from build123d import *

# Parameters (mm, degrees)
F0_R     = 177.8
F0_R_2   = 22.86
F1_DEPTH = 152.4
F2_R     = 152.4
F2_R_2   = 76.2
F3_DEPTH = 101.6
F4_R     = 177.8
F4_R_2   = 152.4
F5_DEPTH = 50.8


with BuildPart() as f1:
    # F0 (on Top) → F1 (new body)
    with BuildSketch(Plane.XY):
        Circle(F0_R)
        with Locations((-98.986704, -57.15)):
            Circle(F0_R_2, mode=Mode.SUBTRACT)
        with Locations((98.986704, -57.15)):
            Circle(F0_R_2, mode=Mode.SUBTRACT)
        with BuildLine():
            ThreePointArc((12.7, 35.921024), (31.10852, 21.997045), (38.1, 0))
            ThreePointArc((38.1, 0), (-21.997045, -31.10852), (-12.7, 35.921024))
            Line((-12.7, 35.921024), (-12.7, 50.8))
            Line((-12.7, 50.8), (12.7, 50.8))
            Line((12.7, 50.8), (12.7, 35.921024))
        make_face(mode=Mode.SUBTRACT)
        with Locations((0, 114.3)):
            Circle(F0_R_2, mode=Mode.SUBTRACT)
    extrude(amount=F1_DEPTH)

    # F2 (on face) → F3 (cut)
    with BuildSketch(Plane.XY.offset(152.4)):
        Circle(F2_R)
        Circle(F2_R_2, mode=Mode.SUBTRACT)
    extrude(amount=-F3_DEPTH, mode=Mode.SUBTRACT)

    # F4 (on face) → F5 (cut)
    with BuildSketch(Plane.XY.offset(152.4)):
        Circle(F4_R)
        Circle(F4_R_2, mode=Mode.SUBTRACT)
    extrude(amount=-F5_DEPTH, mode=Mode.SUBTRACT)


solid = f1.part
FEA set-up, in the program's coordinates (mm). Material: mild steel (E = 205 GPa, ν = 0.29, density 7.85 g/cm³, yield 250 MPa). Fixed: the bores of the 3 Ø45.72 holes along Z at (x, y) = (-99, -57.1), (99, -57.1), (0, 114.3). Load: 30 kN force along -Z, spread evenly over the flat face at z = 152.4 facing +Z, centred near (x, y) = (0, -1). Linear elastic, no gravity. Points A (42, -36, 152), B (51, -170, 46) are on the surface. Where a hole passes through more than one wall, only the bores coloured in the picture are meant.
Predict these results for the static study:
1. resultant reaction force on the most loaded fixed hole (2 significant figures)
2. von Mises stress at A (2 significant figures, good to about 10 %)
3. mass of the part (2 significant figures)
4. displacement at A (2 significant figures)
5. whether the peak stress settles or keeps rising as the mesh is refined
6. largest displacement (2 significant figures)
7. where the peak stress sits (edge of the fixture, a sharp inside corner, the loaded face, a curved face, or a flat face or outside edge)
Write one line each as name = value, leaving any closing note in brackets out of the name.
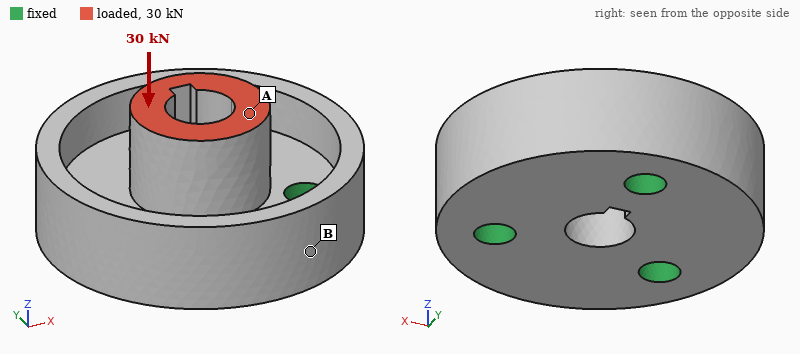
resultant reaction force on the most loaded fixed hole = 10 kN
von Mises stress at A = 2.4 MPa
mass of the part = 57 kg
displacement at A = 2.5 µm
whether the peak stress settles or keeps rising as the mesh is refined = keeps rising
largest displacement = 2.6 µm
where the peak stress sits = edge of the fixture
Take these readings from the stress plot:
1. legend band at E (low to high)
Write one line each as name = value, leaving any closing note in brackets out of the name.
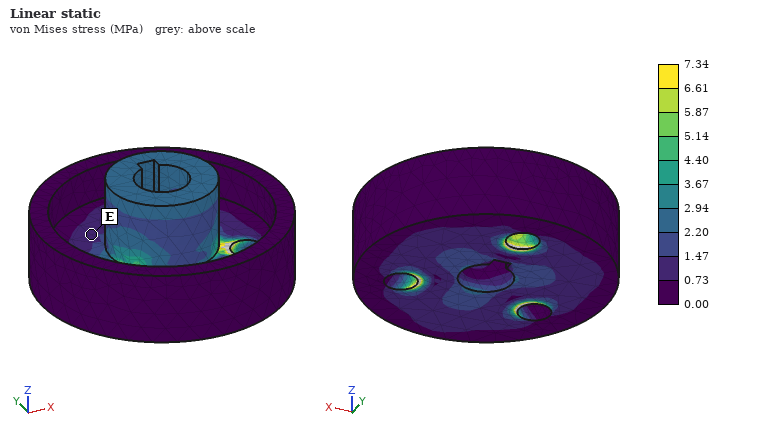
legend band at E = 0.73 to 1.47 MPa
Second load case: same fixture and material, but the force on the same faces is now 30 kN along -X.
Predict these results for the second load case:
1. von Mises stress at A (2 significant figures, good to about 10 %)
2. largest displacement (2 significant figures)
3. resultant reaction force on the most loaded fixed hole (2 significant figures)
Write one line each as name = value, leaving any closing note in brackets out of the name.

von Mises stress at A = 7.2 MPa
largest displacement = 16 µm
resultant reaction force on the most loaded fixed hole = 22 kN
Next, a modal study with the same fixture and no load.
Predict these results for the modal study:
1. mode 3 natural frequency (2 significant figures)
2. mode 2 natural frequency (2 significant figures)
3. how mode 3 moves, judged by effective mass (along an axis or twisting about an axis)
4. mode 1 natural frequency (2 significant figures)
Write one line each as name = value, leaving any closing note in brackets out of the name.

mode 3 natural frequency = 3200 Hz
mode 2 natural frequency = 2500 Hz
how mode 3 moves, judged by effective mass = along Z
mode 1 natural frequency = 2500 Hz
